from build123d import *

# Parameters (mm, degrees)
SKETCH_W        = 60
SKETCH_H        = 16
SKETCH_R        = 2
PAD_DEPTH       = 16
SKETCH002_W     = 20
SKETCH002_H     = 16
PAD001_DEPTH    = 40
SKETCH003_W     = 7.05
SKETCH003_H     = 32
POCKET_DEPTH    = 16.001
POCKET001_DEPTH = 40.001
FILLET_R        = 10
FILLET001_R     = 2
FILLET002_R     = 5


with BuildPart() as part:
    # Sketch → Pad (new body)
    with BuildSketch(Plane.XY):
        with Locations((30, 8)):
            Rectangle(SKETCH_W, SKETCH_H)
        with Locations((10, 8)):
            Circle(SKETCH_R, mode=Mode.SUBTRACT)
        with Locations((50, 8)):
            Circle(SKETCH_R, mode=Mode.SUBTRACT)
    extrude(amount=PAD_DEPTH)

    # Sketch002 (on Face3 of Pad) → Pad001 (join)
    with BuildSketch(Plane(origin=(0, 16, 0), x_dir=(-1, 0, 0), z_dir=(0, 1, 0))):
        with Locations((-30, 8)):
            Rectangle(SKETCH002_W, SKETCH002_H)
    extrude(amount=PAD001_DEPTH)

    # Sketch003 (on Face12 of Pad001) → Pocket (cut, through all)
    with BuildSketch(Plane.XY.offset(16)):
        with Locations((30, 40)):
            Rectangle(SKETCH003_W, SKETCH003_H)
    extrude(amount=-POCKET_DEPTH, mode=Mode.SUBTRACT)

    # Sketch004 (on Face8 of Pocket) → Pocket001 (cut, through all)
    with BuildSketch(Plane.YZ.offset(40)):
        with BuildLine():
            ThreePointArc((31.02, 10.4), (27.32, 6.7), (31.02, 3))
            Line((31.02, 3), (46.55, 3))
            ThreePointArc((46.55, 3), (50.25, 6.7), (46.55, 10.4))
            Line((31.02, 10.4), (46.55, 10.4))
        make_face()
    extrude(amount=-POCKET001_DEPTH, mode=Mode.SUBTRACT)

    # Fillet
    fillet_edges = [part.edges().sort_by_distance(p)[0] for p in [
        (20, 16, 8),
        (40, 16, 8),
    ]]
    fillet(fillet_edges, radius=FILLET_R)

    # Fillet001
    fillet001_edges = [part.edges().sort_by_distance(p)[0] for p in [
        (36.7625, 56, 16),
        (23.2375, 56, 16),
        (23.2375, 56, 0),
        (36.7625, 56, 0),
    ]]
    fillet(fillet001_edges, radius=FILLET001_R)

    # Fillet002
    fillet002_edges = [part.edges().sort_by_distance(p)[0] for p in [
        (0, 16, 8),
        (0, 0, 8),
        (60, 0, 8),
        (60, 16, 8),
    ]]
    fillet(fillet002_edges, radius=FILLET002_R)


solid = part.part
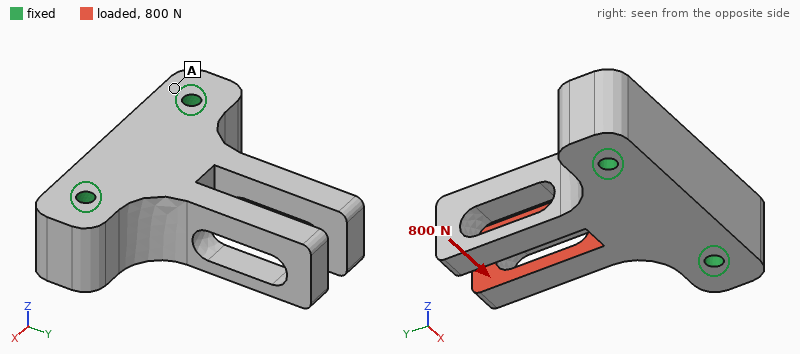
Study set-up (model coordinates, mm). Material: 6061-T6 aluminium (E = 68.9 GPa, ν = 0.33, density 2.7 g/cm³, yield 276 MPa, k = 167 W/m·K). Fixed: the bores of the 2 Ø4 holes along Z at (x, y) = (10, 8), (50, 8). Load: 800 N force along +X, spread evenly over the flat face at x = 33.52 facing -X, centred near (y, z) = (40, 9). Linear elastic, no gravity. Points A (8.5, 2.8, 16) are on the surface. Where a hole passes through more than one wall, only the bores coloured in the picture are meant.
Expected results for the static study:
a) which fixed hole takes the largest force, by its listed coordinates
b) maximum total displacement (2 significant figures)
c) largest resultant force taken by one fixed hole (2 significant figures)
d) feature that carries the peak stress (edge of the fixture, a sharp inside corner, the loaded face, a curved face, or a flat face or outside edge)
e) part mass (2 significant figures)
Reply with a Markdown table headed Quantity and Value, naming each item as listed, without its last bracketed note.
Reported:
| Quantity | Value |
|---|---|
| which fixed hole takes the largest force, by its listed coordinates | (10, 8) |
| maximum total displacement | 0.30 mm |
| largest resultant force taken by one fixed hole | 840 N |
| feature that carries the peak stress | the loaded face |
| part mass | 61 g |
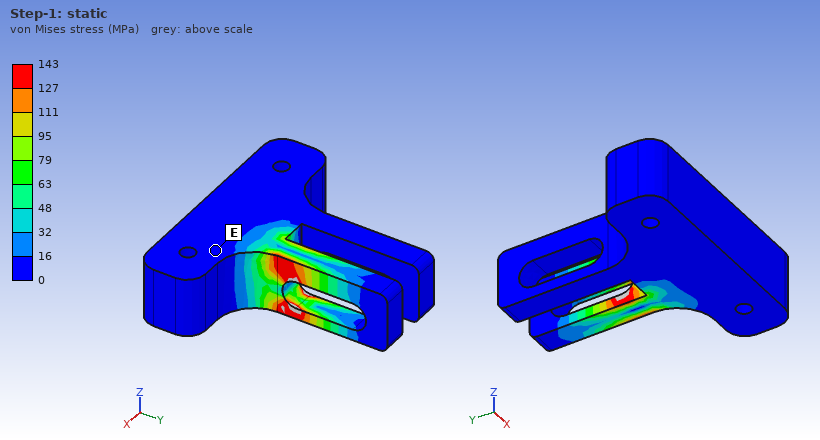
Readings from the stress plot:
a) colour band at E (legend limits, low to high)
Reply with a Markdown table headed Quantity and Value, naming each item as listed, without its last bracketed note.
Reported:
| Quantity | Value |
|---|---|
| colour band at E | 0 to 16 MPa |
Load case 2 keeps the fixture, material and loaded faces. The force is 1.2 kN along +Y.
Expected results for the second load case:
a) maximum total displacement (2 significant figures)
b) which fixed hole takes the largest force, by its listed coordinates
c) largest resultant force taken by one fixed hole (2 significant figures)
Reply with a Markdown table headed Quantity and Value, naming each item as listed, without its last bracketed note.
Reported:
| Quantity | Value |
|---|---|
| maximum total displacement | 0.10 mm |
| which fixed hole takes the largest force, by its listed coordinates | (50, 8) |
| largest resultant force taken by one fixed hole | 770 N |
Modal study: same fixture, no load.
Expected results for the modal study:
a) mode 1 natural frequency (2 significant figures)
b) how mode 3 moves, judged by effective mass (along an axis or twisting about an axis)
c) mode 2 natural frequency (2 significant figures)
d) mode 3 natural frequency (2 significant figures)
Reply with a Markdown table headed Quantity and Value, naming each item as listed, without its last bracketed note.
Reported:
| Quantity | Value |
|---|---|
| mode 1 natural frequency | 4000 Hz |
| how mode 3 moves, judged by effective mass | along Z |
| mode 2 natural frequency | 4000 Hz |
| mode 3 natural frequency | 4700 Hz |
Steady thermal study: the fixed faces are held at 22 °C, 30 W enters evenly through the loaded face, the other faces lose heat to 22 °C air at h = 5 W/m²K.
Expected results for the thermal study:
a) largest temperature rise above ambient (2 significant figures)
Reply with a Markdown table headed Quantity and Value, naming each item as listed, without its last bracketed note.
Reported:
| Quantity | Value |
|---|---|
| largest temperature rise above ambient | 62 K |
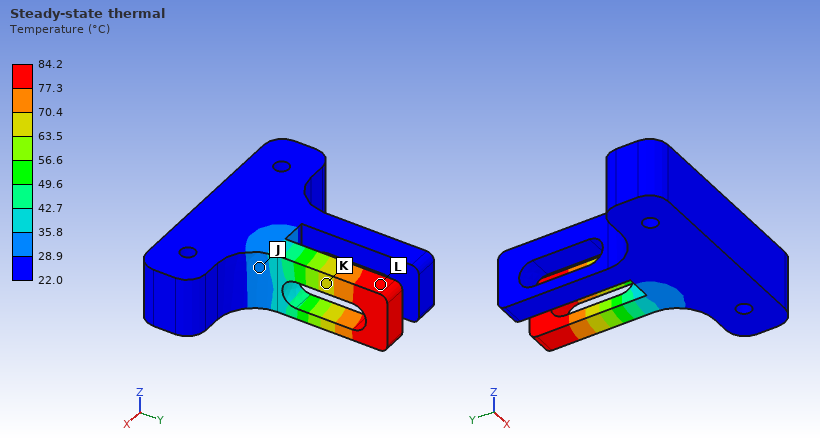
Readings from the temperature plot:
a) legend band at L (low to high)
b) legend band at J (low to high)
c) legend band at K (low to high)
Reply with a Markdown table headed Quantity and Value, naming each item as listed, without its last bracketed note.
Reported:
| Quantity | Value |
|---|---|
| legend band at L | 77.3 to 84.2 °C |
| legend band at J | 28.9 to 35.8 °C |
| legend band at K | 63.5 to 70.4 °C |
